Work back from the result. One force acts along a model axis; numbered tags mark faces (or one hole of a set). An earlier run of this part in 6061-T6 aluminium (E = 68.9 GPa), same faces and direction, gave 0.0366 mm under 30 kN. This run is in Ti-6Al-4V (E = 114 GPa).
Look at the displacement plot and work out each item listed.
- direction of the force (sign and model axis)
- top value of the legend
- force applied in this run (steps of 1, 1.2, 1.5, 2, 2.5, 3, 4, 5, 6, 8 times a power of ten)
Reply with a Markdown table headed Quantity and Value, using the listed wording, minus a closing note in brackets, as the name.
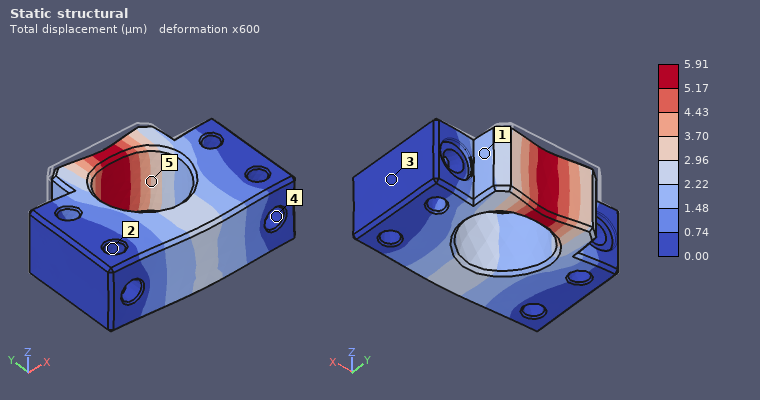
| Quantity | Value |
|---|---|
| direction of the force | -Y |
| top value of the legend | 5.91 µm |
| force applied in this run | 8 kN |
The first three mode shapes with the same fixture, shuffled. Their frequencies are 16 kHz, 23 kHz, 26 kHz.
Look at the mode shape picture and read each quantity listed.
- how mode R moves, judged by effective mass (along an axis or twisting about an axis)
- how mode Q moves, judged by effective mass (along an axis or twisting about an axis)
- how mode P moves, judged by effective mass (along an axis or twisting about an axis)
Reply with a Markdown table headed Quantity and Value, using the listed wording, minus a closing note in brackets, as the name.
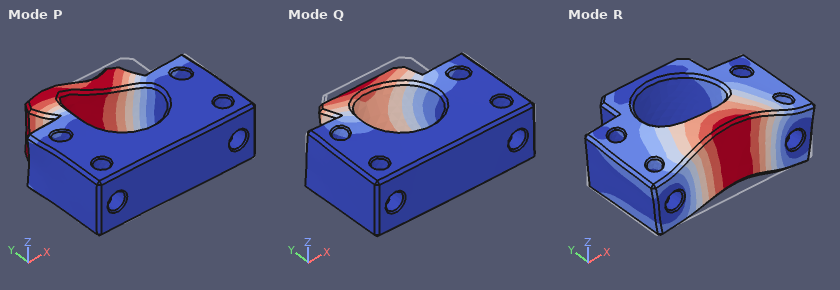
| Quantity | Value |
|---|---|
| how mode R moves, judged by effective mass | along Z |
| how mode Q moves, judged by effective mass | along Z |
| how mode P moves, judged by effective mass | along X |
